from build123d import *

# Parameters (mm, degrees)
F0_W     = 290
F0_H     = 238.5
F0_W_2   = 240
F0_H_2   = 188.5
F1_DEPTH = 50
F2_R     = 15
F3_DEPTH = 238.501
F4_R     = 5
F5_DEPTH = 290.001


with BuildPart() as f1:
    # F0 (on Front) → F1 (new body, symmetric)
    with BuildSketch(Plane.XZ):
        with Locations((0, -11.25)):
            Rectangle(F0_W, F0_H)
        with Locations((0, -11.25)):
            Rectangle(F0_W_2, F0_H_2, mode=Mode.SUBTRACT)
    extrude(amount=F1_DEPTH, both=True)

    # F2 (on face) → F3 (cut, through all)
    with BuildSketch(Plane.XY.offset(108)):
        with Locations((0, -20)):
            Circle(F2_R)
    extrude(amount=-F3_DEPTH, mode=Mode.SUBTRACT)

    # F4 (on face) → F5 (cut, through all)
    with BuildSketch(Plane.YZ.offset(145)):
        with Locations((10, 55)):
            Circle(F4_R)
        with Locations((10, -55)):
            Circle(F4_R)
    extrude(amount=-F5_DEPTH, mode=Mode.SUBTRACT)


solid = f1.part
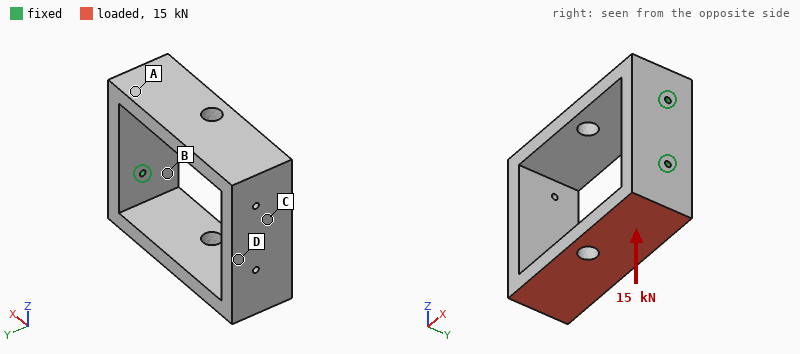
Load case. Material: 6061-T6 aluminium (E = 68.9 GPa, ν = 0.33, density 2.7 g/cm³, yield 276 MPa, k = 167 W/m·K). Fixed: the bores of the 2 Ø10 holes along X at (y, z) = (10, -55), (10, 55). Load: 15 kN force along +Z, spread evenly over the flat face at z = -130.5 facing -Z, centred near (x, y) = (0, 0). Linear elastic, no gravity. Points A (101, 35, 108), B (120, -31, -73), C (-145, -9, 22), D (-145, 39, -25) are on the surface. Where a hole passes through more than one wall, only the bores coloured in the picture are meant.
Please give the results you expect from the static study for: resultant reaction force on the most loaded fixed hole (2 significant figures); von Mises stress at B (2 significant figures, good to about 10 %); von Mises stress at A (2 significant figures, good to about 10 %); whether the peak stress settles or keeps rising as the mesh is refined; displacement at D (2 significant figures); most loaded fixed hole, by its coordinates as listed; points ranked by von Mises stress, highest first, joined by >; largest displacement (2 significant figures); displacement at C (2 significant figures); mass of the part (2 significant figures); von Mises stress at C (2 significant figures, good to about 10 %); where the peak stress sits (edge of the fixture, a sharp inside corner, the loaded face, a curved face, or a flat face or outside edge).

14 kN
65 MPa
42 MPa
keeps rising
1.6 mm
(10, -55)
B > A > C > D
1.6 mm
1.6 mm
6.3 kg
18 MPa
edge of the fixture
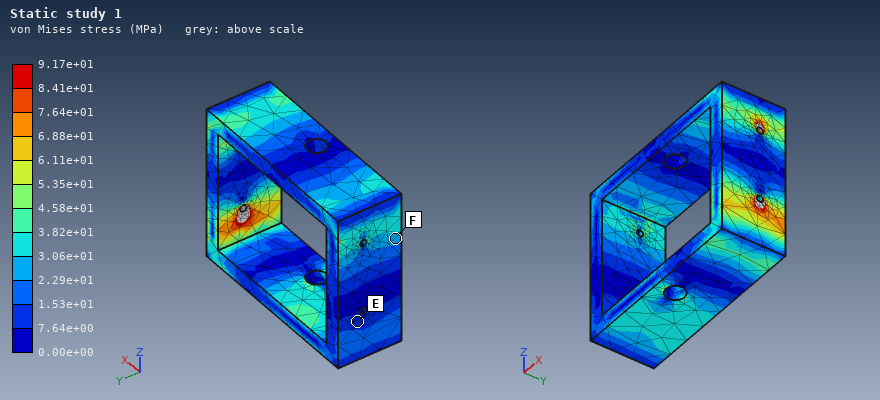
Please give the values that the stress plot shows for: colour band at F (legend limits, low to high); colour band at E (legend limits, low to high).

2.29e+01 to 3.06e+01 MPa
7.64e+00 to 1.53e+01 MPa
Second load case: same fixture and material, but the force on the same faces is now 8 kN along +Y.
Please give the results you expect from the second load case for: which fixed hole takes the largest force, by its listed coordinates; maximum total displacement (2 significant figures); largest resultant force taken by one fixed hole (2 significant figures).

(10, -55)
1.2 mm
13 kN
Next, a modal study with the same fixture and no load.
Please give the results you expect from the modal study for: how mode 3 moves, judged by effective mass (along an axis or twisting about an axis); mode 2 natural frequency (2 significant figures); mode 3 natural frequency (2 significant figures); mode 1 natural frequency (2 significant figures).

twisting about X
220 Hz
490 Hz
210 Hz
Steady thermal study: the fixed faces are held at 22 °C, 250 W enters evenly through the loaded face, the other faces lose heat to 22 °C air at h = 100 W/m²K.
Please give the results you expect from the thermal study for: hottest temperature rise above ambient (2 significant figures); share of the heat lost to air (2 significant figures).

27 K
71 %
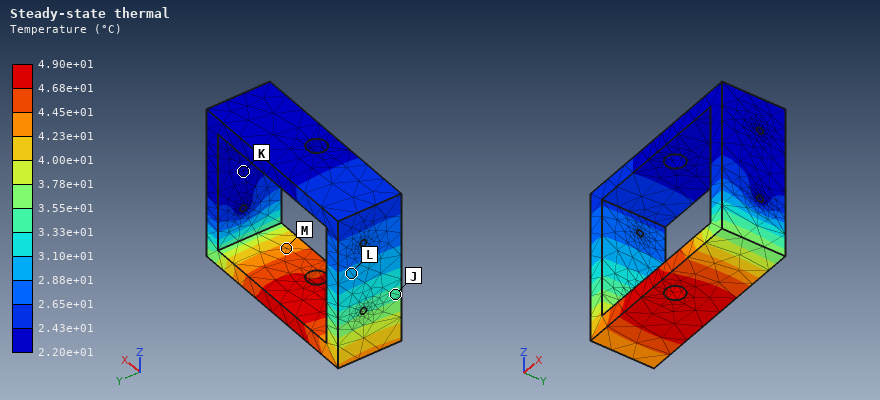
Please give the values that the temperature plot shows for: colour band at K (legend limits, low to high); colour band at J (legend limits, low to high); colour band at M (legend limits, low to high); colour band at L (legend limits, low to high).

2.20e+01 to 2.43e+01 °C
3.33e+01 to 3.55e+01 °C
4.23e+01 to 4.45e+01 °C
2.88e+01 to 3.10e+01 °C
